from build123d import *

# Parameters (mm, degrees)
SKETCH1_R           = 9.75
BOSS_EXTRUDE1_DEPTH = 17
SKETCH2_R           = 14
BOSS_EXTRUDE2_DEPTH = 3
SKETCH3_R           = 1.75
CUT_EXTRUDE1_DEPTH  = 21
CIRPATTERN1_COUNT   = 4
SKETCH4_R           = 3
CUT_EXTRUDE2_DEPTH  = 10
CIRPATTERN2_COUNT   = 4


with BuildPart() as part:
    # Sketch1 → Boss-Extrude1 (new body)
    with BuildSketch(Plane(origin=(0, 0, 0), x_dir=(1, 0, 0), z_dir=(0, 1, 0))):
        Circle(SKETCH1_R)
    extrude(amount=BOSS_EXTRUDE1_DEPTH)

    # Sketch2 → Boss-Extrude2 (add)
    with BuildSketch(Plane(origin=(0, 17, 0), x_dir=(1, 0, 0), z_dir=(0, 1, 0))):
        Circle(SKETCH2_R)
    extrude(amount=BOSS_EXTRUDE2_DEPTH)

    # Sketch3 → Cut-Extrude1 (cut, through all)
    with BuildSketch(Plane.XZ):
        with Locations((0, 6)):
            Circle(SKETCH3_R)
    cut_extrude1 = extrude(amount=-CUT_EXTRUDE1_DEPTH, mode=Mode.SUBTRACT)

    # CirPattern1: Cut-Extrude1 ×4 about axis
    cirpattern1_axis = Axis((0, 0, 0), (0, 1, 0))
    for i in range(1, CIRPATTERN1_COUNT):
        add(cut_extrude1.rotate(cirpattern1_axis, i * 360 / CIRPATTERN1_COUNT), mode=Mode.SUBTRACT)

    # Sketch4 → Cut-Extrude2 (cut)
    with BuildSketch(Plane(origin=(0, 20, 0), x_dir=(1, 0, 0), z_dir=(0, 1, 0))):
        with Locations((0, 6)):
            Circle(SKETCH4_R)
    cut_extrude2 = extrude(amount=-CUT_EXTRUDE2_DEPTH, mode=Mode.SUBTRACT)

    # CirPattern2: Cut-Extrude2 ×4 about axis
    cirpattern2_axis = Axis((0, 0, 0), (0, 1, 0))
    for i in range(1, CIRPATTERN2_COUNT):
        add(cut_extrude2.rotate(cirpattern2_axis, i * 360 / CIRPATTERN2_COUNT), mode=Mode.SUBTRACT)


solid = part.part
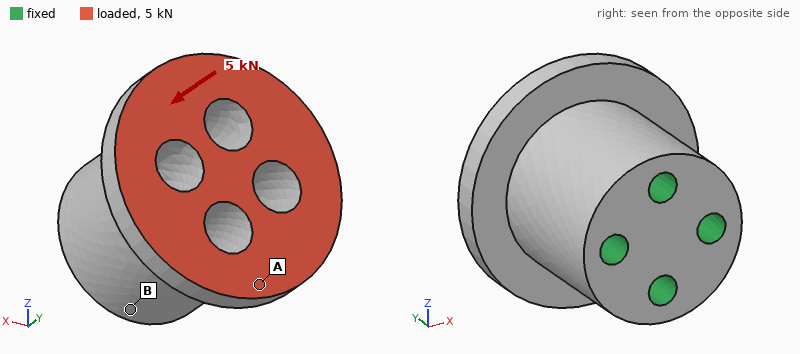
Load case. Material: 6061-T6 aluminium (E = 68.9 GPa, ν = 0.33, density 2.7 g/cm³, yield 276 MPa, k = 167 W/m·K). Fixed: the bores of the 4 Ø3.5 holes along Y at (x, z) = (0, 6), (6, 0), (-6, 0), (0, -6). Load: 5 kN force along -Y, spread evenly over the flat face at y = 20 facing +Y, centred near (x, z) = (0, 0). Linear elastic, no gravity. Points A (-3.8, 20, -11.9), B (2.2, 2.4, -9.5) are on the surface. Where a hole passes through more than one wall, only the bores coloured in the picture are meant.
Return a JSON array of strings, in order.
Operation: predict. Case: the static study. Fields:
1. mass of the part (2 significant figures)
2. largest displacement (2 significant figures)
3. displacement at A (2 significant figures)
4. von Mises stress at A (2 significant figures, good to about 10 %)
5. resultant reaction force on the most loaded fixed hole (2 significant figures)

["15 g", "23 µm", "18 µm", "37 MPa", "1.3 kN"]
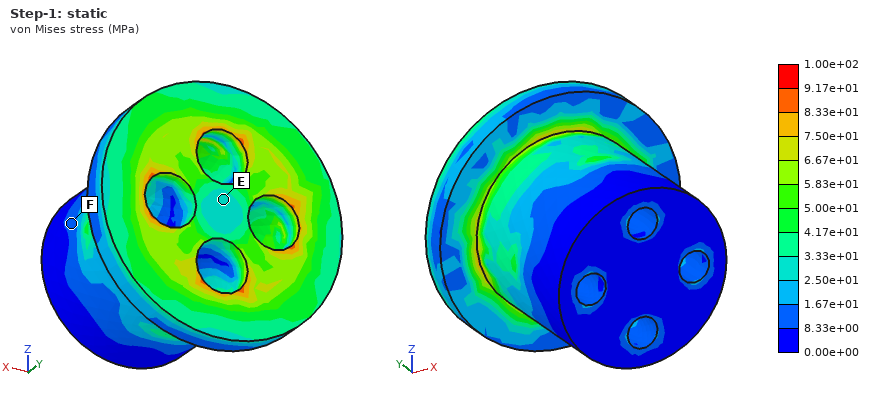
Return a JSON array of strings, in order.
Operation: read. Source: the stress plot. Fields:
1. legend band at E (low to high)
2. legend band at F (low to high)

["2.50e+01 to 3.33e+01 MPa", "8.33e+00 to 1.67e+01 MPa"]
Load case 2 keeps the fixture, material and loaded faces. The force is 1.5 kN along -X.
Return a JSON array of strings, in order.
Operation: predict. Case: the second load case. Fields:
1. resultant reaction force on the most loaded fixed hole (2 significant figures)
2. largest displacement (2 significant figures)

["1.1 kN", "17 µm"]
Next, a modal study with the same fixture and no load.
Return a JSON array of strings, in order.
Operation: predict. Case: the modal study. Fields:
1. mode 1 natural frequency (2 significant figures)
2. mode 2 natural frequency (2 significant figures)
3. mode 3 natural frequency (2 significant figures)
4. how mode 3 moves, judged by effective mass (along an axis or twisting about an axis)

["28 kHz", "28 kHz", "31 kHz", "twisting about Y"]
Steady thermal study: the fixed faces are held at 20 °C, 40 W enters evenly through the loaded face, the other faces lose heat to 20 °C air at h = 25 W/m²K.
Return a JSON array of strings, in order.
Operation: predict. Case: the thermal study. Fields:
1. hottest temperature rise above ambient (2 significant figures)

["17 K"]
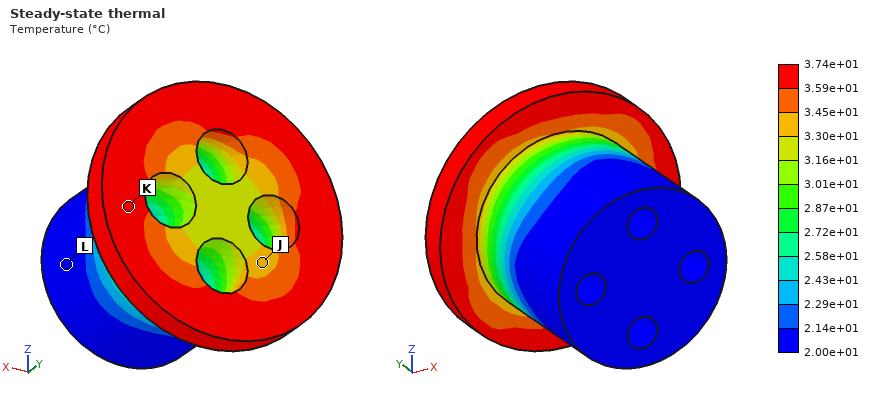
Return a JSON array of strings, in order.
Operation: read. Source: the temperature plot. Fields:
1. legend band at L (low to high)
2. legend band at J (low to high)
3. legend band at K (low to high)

["2.00e+01 to 2.14e+01 °C", "3.30e+01 to 3.45e+01 °C", "3.59e+01 to 3.74e+01 °C"]
